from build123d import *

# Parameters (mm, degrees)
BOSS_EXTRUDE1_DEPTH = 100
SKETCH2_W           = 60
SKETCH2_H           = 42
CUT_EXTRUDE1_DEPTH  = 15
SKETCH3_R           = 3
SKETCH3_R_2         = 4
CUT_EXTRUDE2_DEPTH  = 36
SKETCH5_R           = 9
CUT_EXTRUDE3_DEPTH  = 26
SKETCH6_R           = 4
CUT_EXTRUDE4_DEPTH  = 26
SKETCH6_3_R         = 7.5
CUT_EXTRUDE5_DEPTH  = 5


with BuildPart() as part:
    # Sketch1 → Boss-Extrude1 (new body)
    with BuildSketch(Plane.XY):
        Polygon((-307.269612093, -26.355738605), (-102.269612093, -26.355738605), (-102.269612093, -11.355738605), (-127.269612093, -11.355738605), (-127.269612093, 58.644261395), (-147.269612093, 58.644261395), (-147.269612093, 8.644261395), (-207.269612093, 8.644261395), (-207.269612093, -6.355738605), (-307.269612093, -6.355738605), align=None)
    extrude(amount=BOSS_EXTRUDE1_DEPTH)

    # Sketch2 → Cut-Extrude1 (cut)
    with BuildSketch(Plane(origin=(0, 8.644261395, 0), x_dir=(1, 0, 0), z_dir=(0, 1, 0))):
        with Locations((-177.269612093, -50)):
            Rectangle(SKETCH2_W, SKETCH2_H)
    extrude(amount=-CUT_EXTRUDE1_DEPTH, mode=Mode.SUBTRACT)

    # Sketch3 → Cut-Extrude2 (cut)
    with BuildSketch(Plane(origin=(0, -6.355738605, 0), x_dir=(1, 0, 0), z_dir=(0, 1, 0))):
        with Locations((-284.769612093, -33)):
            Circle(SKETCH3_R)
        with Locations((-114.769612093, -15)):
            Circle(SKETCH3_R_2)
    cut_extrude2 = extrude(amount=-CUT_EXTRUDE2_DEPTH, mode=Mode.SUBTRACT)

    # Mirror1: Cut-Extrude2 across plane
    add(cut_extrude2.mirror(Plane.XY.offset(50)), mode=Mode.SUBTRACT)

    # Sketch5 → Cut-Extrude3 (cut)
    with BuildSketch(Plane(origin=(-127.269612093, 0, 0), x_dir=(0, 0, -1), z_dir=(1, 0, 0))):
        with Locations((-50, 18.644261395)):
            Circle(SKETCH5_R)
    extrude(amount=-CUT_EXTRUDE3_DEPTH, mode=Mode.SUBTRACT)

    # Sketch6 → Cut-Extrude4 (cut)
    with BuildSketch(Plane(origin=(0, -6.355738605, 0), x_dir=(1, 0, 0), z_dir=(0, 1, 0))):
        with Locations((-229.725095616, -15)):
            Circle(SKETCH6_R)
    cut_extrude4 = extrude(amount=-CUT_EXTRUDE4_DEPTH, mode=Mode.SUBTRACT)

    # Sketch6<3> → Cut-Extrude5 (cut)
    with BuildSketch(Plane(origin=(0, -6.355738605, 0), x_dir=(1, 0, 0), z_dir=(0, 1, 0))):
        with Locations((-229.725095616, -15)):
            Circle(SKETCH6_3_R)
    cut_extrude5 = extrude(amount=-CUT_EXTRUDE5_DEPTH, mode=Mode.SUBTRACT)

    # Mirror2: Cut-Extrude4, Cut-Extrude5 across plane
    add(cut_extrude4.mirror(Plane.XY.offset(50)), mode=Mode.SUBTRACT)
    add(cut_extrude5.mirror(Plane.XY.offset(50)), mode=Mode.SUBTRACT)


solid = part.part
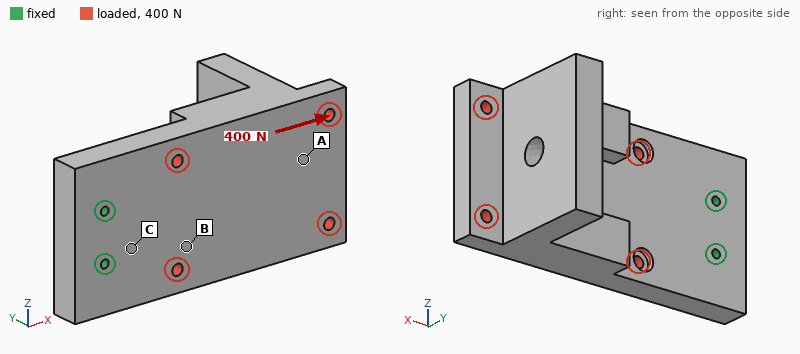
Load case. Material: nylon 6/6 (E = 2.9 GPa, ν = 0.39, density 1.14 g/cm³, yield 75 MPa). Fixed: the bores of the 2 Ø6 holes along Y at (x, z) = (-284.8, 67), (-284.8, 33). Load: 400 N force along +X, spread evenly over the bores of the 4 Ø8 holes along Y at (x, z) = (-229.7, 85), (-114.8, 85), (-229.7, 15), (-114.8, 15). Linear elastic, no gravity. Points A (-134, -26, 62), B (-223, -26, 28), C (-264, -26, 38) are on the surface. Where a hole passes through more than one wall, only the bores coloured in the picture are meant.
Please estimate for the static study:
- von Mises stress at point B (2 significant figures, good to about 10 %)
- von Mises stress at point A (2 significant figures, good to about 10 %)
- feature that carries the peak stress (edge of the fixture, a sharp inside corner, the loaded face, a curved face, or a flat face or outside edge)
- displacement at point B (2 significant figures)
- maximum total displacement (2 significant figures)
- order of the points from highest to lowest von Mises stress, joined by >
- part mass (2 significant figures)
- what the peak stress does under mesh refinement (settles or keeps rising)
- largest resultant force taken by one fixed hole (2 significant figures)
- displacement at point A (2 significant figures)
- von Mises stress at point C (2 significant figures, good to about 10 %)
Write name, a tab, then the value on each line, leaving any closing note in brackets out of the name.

von Mises stress at point B	0.28 MPa
von Mises stress at point A	0.11 MPa
feature that carries the peak stress	edge of the fixture
displacement at point B	16 µm
maximum total displacement	71 µm
order of the points from highest to lowest von Mises stress, joined by >	C > B > A
part mass	650 g
what the peak stress does under mesh refinement	keeps rising
largest resultant force taken by one fixed hole	200 N
displacement at point A	54 µm
von Mises stress at point C	0.42 MPa
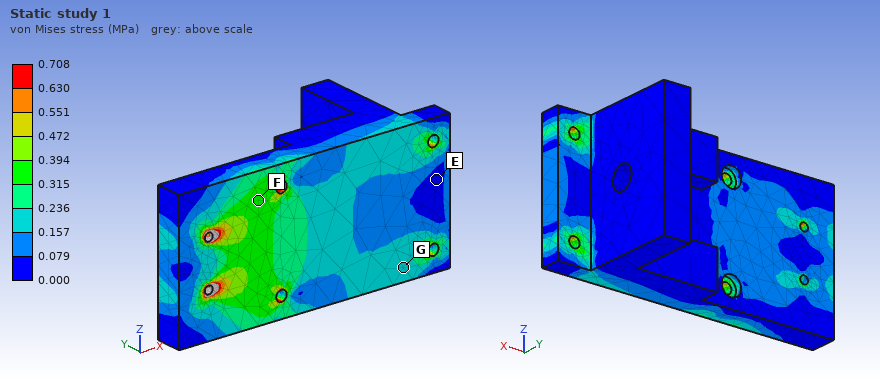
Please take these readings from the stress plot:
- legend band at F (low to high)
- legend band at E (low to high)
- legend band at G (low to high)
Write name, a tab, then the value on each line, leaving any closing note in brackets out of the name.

legend band at F	0.315 to 0.394 MPa
legend band at E	0.000 to 0.079 MPa
legend band at G	0.157 to 0.236 MPa
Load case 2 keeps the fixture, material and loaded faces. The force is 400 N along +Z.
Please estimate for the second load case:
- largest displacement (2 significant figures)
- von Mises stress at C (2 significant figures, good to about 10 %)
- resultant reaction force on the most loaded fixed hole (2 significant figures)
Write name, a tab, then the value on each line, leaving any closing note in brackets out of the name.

largest displacement	0.28 mm
von Mises stress at C	1.5 MPa
resultant reaction force on the most loaded fixed hole	1.2 kN
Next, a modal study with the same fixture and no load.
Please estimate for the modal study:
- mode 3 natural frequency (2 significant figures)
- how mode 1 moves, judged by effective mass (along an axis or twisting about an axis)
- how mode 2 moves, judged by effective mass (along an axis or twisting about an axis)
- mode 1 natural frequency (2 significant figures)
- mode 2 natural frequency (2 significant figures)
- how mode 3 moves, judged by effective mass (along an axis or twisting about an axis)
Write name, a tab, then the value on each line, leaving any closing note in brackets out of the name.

mode 3 natural frequency	390 Hz
how mode 1 moves, judged by effective mass	along Y
how mode 2 moves, judged by effective mass	along Z
mode 1 natural frequency	100 Hz
mode 2 natural frequency	260 Hz
how mode 3 moves, judged by effective mass	along Z
